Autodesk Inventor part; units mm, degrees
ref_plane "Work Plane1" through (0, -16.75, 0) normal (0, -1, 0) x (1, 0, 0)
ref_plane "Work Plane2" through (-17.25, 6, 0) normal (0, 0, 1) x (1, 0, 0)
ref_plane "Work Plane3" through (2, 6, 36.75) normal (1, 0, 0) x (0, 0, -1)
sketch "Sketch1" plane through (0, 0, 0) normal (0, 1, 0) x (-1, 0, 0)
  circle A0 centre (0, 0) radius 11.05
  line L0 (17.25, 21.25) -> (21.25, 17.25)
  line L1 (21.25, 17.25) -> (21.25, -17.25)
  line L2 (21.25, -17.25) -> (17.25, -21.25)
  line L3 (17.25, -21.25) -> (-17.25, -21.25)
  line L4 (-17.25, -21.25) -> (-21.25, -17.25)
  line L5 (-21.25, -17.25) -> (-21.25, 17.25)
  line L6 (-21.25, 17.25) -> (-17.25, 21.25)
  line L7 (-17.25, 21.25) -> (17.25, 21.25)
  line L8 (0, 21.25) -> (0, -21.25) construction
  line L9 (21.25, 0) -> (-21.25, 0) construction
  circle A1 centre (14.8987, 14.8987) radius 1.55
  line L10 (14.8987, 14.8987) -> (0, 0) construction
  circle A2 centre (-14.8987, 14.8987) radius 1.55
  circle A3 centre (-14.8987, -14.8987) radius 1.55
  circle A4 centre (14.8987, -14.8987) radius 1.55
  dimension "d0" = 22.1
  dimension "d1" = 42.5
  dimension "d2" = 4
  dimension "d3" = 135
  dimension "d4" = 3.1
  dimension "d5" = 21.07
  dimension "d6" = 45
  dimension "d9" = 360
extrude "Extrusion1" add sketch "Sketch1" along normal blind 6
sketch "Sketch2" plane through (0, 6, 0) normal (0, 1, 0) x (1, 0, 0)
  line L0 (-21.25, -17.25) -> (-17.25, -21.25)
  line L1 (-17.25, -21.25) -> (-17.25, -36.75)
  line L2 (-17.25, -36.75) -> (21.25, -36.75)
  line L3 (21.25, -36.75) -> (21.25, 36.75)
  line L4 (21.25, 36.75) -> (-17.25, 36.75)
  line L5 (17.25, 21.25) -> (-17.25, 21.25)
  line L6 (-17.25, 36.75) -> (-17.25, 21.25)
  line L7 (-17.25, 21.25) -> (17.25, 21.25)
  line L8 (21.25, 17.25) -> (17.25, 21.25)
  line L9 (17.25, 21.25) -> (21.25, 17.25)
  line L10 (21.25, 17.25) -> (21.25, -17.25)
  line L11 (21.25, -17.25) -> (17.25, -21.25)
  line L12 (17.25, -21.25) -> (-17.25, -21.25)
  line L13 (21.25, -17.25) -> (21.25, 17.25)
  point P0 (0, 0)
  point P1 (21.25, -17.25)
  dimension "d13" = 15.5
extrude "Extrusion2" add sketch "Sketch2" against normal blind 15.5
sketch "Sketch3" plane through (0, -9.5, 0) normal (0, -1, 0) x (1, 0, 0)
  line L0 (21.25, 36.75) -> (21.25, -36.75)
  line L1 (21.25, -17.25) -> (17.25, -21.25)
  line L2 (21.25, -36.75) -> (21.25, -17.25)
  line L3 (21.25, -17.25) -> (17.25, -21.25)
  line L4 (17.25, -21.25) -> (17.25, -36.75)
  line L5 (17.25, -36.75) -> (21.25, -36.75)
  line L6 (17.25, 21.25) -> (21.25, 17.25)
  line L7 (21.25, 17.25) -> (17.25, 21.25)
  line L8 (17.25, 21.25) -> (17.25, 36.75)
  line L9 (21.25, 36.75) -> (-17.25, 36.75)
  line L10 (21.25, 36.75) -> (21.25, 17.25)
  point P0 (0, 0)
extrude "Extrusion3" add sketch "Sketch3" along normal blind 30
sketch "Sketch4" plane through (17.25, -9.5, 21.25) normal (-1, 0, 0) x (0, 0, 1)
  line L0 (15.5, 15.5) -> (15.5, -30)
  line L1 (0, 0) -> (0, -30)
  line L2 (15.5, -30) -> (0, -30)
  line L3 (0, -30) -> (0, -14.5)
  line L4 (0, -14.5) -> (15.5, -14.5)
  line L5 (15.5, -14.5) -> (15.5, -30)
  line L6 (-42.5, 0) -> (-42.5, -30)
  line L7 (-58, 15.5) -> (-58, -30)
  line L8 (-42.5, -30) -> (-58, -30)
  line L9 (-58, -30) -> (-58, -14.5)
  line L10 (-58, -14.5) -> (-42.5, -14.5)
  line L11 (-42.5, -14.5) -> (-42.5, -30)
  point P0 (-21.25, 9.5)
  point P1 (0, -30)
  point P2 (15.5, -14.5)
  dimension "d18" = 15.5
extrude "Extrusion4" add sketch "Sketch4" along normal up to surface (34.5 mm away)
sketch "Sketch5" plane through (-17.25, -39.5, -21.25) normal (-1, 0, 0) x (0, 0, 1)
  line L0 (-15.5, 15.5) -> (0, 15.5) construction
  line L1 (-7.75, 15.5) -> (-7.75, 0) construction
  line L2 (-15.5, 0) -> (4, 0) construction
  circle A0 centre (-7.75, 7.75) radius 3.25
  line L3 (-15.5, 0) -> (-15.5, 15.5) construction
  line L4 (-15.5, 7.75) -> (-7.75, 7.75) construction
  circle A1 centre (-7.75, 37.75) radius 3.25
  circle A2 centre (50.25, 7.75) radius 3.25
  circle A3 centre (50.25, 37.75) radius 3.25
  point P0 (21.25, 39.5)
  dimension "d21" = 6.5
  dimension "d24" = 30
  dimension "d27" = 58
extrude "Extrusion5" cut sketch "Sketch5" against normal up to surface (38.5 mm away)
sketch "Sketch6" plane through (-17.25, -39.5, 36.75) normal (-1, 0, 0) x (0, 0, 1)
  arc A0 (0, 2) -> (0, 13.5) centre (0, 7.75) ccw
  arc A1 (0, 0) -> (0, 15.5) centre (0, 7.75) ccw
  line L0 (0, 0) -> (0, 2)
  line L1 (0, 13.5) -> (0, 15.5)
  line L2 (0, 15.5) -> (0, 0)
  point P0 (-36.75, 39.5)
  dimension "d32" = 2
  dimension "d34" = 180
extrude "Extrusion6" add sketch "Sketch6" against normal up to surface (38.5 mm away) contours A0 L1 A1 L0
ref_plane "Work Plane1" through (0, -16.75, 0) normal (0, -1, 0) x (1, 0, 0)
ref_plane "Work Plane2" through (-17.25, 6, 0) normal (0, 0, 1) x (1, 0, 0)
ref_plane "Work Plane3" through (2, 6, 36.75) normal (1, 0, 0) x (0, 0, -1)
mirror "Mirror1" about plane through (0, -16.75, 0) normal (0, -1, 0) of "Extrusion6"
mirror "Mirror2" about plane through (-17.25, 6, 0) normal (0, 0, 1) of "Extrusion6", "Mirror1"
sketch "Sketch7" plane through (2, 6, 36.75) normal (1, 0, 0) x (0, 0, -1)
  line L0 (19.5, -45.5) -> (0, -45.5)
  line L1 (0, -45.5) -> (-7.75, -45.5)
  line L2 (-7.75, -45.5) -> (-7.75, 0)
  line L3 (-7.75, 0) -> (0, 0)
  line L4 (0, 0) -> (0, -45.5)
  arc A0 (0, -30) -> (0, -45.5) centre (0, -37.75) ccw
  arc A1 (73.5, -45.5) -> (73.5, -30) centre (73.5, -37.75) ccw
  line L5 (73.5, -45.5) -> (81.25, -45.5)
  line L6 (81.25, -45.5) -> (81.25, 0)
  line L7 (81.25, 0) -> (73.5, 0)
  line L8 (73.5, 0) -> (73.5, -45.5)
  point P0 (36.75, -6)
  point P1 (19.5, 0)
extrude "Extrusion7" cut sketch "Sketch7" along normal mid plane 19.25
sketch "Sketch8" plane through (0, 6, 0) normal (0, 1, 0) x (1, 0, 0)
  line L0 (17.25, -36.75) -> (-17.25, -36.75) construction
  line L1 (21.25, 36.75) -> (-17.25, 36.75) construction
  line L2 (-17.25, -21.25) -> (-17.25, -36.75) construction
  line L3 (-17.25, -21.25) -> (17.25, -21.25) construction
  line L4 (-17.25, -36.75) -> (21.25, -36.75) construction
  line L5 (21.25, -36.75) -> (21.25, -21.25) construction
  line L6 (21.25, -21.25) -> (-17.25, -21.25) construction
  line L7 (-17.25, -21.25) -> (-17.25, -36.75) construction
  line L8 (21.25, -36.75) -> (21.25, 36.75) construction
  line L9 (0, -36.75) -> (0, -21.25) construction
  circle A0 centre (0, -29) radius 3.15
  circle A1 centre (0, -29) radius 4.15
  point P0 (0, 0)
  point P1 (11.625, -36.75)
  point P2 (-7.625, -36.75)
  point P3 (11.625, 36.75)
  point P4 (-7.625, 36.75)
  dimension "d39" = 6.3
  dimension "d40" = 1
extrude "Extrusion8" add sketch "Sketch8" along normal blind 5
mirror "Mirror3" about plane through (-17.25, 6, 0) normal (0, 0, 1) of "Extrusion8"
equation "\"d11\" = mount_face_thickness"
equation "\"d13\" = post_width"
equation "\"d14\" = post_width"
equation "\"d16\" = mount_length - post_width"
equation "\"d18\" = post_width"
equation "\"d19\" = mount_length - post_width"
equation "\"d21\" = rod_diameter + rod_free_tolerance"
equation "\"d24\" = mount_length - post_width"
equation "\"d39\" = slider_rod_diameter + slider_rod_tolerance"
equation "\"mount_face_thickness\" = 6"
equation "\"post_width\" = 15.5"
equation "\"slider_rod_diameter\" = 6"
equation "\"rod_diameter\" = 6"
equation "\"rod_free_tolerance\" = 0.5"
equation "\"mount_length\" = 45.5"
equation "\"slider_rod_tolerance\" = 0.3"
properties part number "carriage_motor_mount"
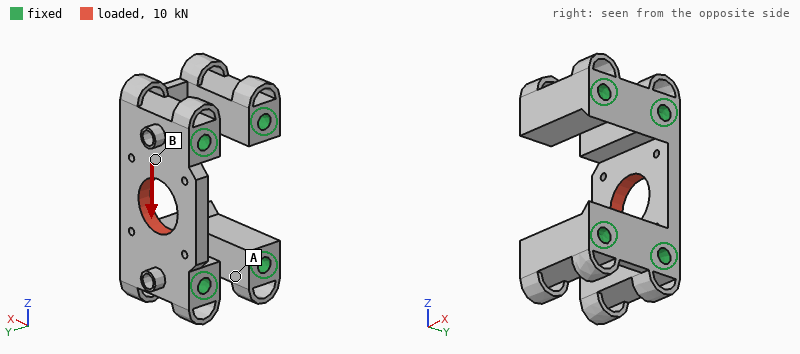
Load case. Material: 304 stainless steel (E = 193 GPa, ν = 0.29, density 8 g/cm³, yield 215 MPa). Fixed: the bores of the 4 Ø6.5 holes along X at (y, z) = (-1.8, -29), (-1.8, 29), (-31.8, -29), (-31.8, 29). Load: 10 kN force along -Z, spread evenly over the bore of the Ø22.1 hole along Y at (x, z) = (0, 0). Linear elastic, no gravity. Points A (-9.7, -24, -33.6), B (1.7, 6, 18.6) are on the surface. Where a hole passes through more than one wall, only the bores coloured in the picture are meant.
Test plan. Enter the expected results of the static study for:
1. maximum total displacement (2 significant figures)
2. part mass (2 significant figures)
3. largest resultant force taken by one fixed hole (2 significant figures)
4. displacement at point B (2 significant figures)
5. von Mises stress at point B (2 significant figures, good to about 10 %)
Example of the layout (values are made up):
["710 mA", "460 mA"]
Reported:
["4.1 µm", "370 g", "5.0 kN", "1.7 µm", "19 MPa"]
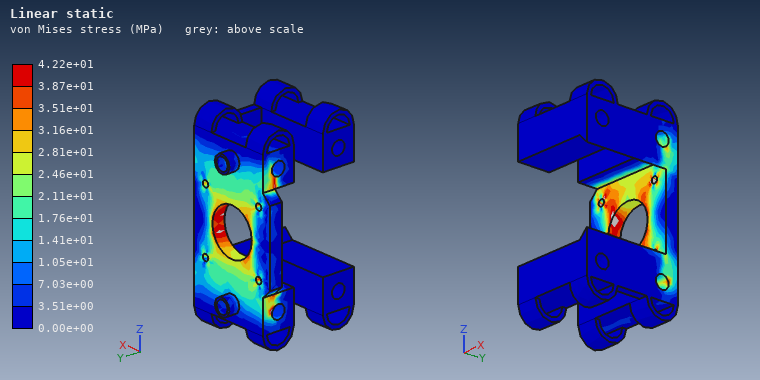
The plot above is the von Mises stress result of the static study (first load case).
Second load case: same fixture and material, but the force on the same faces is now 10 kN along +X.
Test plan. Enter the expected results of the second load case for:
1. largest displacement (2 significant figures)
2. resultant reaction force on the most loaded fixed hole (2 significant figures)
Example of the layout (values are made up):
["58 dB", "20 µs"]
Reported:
["9.5 µm", "5.0 kN"]
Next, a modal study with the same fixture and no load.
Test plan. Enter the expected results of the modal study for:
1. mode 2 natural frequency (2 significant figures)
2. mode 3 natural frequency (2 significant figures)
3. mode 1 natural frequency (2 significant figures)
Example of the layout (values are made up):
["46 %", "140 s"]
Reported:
["14 kHz", "25 kHz", "12 kHz"]
